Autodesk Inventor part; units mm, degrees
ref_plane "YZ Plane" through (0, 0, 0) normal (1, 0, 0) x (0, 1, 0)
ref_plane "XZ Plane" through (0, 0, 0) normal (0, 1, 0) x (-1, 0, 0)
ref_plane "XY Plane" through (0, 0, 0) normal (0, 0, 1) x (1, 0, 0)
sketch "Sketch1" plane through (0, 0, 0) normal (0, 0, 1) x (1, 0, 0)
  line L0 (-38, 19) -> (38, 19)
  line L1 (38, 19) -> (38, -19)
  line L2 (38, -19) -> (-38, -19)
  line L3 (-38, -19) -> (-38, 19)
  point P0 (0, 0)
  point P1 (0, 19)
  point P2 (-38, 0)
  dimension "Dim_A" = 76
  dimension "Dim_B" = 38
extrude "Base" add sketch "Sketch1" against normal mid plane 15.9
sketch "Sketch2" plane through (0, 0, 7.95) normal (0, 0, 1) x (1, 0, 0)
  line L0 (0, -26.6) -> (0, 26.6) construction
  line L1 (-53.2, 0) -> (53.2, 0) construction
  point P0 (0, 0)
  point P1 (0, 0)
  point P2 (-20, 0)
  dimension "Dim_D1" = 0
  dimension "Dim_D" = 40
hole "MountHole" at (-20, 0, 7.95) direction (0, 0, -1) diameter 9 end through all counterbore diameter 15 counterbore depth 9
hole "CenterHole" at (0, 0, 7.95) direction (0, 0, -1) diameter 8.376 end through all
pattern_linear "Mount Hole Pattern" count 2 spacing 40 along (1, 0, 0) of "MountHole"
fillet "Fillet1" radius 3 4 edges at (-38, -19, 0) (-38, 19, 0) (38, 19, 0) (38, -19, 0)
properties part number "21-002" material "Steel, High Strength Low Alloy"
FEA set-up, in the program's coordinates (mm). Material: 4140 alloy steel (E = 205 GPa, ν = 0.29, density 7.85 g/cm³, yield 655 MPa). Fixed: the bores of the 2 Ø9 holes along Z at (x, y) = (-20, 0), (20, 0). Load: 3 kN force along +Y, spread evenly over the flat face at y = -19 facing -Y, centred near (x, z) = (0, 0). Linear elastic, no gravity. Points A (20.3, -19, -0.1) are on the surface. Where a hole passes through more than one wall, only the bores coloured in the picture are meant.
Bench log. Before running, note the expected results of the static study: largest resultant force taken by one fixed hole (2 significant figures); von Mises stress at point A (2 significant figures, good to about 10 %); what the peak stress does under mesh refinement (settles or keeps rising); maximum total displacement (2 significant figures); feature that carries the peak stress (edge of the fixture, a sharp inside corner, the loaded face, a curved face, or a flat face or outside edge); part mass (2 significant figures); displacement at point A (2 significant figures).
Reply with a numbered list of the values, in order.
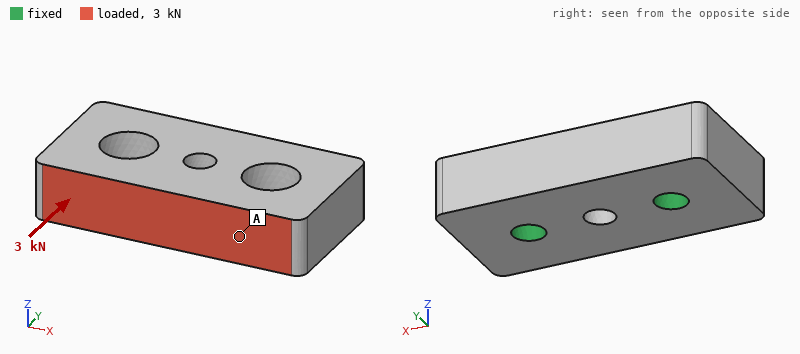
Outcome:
1. 1.5 kN
2. 3.0 MPa
3. keeps rising
4. 2.4 µm
5. edge of the fixture
6. 320 g
7. 1.8 µm
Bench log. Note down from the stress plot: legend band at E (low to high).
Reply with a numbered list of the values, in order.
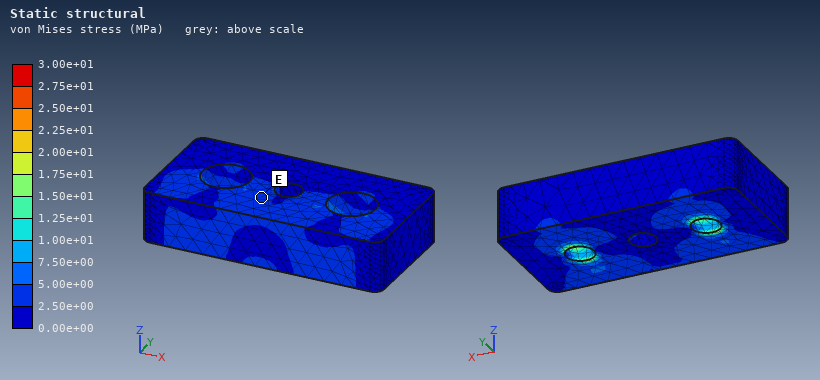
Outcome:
1. 2.50e+00 to 5.00e+00 MPa
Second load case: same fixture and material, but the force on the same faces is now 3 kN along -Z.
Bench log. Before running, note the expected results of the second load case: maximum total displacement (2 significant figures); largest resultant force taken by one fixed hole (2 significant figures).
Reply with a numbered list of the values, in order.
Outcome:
1. 9.5 µm
2. 1.5 kN
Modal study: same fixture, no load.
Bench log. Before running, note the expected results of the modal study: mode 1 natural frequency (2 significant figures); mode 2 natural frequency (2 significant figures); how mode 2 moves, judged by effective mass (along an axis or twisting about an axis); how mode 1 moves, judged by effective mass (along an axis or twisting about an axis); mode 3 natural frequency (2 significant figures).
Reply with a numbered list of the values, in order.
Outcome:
1. 9100 Hz
2. 14 kHz
3. twisting about Z
4. along Y
5. 16 kHz
